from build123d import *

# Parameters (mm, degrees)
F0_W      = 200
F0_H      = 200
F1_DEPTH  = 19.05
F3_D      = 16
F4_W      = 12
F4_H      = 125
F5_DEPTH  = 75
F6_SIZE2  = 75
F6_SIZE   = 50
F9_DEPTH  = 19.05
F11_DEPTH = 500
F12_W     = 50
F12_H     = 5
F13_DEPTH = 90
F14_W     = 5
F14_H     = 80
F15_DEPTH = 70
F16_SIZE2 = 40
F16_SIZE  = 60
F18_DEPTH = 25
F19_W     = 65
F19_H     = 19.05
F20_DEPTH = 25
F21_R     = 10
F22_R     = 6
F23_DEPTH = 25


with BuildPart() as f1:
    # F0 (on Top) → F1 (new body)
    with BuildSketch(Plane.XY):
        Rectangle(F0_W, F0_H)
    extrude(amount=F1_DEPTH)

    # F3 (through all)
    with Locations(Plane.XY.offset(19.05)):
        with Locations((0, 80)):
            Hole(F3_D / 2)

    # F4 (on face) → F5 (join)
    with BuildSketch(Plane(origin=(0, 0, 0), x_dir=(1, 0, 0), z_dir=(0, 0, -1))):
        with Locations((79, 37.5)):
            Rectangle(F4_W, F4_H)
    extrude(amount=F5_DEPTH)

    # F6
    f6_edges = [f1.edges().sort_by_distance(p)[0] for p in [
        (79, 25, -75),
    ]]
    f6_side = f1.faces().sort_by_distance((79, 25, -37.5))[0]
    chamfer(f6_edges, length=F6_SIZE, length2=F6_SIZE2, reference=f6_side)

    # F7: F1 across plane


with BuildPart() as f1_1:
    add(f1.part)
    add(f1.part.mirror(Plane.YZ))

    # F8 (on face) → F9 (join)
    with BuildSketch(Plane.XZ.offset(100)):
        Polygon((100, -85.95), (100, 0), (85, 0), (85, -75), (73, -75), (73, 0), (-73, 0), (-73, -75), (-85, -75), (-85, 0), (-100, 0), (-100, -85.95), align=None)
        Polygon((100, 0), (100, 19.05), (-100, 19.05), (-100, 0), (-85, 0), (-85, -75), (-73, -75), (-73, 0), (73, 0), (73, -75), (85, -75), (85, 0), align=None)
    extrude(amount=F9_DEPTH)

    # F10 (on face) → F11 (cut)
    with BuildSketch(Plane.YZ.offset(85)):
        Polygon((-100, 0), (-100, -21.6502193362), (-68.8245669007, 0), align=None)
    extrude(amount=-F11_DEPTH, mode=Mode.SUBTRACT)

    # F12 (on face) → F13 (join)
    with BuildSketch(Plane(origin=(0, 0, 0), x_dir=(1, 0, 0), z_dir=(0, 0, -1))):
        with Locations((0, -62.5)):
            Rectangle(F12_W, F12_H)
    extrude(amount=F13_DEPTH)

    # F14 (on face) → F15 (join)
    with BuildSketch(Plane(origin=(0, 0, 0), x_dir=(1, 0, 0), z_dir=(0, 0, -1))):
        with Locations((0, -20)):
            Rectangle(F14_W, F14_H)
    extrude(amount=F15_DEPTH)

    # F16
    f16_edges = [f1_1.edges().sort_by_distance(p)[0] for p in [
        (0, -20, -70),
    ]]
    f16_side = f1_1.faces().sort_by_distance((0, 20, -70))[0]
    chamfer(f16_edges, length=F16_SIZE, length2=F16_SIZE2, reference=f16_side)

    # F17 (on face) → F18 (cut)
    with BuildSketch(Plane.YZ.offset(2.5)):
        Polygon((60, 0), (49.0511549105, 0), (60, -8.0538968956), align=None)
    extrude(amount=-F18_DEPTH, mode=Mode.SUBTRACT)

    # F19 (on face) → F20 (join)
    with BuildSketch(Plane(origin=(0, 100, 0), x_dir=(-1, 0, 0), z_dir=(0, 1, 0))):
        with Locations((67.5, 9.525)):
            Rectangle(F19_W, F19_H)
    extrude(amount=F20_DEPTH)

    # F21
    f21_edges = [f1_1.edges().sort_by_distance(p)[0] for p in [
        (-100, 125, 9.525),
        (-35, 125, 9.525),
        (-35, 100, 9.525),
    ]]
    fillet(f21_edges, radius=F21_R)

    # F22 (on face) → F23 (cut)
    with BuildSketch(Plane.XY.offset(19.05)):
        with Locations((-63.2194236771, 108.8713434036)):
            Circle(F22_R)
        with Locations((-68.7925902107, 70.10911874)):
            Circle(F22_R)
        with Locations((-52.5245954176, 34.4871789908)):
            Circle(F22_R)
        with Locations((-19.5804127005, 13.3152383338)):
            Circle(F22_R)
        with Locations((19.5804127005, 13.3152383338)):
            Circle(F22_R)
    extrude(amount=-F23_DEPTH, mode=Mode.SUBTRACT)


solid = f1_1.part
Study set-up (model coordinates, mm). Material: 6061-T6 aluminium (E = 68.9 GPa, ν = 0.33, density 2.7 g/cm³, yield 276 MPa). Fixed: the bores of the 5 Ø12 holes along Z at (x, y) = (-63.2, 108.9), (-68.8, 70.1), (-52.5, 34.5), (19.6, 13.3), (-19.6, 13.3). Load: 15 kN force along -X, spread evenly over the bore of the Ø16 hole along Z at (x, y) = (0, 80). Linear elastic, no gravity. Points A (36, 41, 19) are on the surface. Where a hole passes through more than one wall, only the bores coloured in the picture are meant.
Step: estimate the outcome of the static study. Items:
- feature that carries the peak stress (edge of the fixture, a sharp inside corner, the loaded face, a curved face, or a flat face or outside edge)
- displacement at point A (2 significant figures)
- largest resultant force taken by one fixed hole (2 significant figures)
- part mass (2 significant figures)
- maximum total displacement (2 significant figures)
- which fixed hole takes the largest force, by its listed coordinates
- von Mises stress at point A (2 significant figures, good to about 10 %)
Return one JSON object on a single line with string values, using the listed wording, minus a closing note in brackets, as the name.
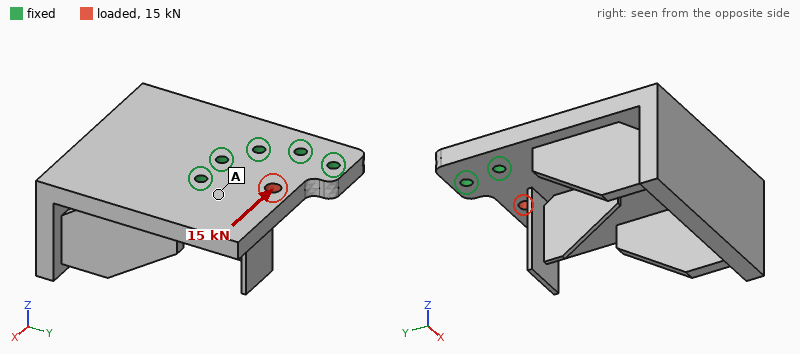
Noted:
{"feature that carries the peak stress": "the loaded face", "displacement at point A": "5.0 µm", "largest resultant force taken by one fixed hole": "5.3 kN", "part mass": "3.8 kg", "maximum total displacement": "16 µm", "which fixed hole takes the largest force, by its listed coordinates": "(-68.8, 70.1)", "von Mises stress at point A": "3.1 MPa"}
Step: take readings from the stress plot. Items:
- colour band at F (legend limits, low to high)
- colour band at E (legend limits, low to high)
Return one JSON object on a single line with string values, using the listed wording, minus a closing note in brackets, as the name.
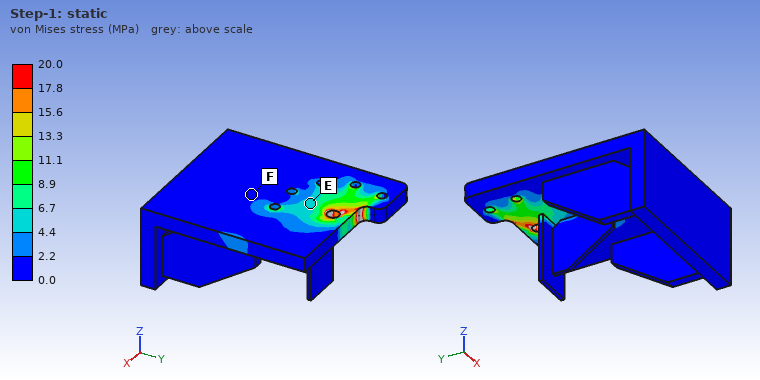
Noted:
{"colour band at F": "0.0 to 2.2 MPa", "colour band at E": "4.4 to 6.7 MPa"}
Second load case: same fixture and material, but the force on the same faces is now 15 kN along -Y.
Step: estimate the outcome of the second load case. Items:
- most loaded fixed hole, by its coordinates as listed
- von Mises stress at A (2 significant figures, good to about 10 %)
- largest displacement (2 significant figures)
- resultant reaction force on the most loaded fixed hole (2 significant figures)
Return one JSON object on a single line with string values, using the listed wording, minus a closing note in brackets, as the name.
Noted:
{"most loaded fixed hole, by its coordinates as listed": "(19.6, 13.3)", "von Mises stress at A": "5.0 MPa", "largest displacement": "16 µm", "resultant reaction force on the most loaded fixed hole": "7.2 kN"}
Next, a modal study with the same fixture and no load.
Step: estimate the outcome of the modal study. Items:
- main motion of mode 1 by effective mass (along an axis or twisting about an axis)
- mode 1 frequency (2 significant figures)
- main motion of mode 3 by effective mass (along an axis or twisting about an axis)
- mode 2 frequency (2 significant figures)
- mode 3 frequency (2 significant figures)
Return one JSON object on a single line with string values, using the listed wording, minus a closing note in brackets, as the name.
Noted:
{"main motion of mode 1 by effective mass": "along Z", "mode 1 frequency": "500 Hz", "main motion of mode 3 by effective mass": "along Z", "mode 2 frequency": "660 Hz", "mode 3 frequency": "1600 Hz"}
